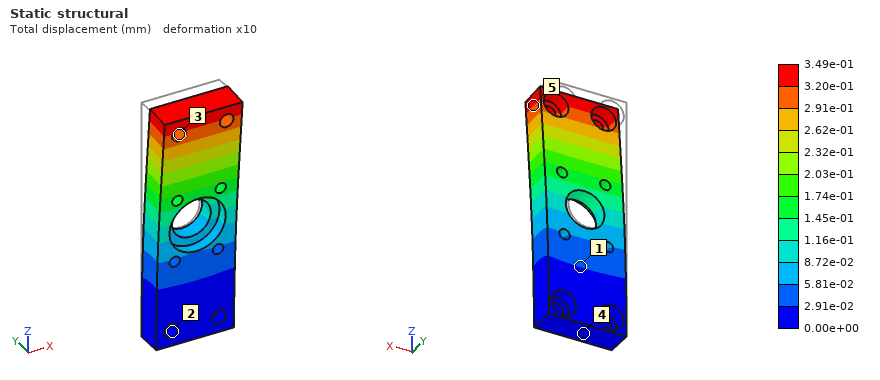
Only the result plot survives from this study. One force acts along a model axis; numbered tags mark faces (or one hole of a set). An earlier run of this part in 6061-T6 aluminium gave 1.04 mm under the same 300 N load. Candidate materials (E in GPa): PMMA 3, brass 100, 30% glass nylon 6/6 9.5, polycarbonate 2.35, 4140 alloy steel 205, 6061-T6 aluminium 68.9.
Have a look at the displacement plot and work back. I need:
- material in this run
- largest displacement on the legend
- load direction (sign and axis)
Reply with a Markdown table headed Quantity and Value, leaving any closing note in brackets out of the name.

| Quantity | Value |
|---|---|
| material in this run | 4140 alloy steel |
| largest displacement on the legend | 3.49e-01 mm |
| load direction | -Y |
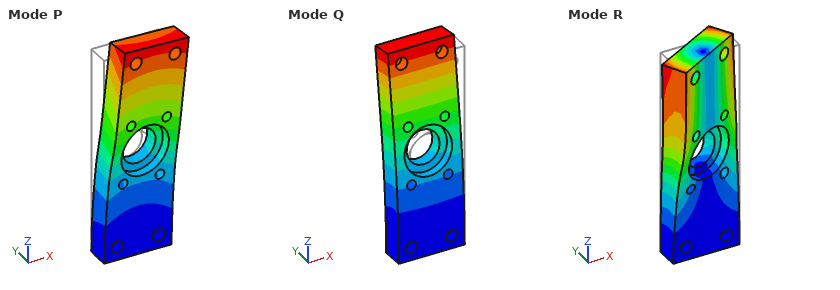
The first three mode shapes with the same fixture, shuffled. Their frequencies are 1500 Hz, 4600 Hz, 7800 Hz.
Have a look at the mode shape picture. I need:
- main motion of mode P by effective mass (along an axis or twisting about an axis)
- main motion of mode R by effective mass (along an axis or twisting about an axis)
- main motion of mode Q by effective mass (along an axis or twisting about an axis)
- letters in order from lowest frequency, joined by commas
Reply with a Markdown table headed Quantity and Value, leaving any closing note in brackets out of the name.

| Quantity | Value |
|---|---|
| main motion of mode P by effective mass | along X |
| main motion of mode R by effective mass | twisting about Z |
| main motion of mode Q by effective mass | along Y |
| letters in order from lowest frequency, joined by commas | Q, P, R |
